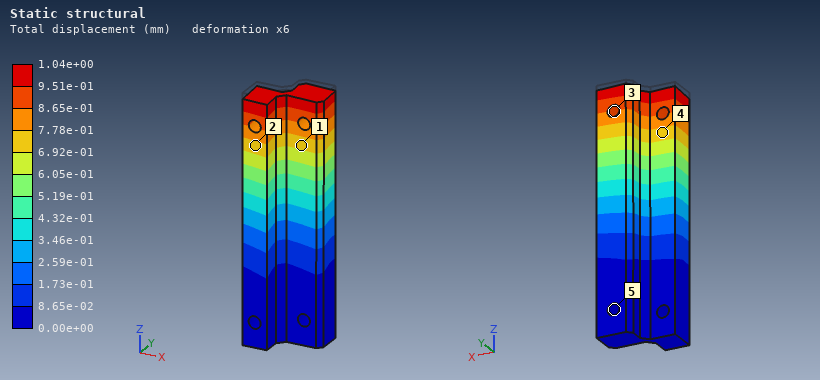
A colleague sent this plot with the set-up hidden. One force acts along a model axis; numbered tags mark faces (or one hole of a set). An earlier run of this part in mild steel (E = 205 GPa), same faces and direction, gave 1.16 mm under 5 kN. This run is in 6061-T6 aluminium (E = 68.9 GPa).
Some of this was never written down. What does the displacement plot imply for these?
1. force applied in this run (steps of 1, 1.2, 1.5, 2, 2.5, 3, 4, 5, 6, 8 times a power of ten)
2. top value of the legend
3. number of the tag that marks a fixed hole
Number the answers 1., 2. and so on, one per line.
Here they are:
1. 1.5 kN
2. 1.04e+00 mm
3. 5
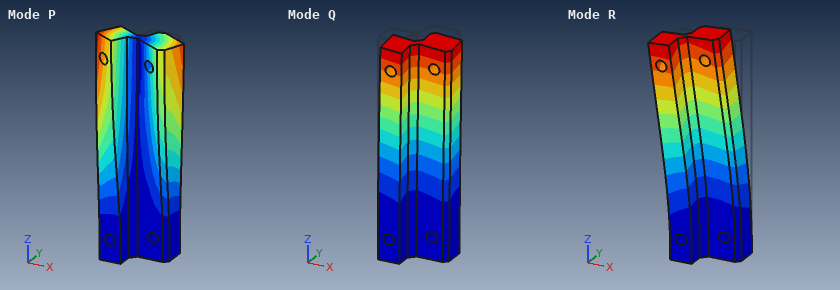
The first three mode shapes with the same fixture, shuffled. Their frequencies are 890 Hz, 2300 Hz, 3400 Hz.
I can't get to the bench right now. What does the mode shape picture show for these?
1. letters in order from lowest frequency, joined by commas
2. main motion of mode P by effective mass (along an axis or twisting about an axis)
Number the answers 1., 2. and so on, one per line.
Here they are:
1. Q, R, P
2. twisting about Z
